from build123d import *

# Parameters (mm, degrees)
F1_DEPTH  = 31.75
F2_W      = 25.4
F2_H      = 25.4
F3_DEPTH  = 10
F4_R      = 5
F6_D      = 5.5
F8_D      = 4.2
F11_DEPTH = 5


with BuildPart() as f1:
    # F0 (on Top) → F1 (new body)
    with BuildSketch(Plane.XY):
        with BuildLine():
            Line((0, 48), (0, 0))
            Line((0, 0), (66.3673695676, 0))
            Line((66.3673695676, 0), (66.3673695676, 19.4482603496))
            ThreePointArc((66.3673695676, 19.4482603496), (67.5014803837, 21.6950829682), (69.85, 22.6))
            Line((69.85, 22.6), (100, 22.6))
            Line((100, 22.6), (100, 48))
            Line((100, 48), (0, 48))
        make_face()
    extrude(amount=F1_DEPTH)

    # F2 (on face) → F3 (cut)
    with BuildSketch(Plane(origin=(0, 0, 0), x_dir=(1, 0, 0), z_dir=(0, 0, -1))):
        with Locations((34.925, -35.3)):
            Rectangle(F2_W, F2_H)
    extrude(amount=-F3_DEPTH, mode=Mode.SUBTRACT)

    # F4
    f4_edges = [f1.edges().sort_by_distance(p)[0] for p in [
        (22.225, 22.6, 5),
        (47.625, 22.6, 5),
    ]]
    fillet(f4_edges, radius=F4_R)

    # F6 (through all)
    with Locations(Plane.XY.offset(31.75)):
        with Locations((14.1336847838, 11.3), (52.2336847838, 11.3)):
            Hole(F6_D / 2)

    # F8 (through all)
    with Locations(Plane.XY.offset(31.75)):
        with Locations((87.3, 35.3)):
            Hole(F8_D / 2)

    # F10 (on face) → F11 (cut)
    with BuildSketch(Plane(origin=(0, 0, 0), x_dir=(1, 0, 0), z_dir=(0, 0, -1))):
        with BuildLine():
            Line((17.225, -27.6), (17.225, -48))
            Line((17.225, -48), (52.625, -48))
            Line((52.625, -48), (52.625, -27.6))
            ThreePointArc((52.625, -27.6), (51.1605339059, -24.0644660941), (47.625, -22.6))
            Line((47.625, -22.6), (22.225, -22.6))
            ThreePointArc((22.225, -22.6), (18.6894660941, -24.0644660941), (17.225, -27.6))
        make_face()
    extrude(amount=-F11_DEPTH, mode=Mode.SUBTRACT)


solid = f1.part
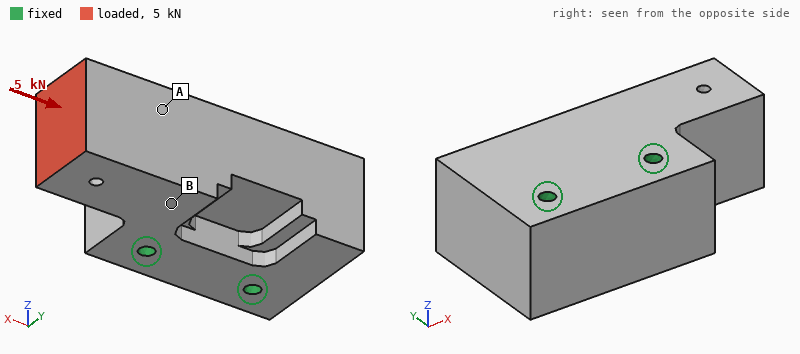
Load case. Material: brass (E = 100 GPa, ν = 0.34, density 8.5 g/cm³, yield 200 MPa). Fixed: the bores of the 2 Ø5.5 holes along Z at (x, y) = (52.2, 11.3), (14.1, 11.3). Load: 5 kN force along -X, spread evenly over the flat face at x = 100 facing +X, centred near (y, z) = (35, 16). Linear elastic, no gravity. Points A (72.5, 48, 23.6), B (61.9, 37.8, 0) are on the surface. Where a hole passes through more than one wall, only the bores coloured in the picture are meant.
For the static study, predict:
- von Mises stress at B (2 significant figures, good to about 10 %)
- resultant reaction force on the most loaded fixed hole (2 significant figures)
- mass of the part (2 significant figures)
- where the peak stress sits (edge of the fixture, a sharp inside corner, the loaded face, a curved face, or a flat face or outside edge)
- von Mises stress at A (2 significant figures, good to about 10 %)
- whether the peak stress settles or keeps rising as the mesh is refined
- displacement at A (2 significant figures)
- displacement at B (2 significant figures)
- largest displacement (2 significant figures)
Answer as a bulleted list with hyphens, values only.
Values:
- 2.9 MPa
- 3.9 kN
- 1.0 kg
- edge of the fixture
- 7.7 MPa
- keeps rising
- 8.0 µm
- 6.4 µm
- 14 µm
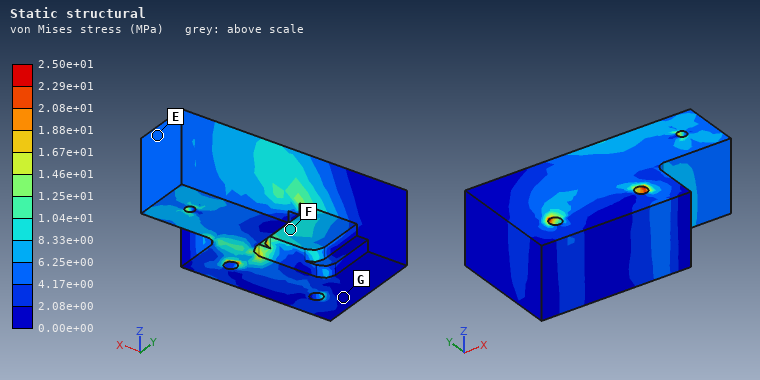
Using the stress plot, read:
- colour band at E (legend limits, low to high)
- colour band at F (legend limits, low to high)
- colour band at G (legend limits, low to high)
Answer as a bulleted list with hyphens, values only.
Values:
- 4.17e+00 to 6.25e+00 MPa
- 8.33e+00 to 1.04e+01 MPa
- 0.00e+00 to 2.08e+00 MPa
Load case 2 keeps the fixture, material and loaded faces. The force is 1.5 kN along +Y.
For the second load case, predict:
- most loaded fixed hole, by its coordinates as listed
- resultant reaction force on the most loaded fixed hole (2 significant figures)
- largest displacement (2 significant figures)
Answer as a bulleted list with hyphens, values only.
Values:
- (52.2, 11.3)
- 3.3 kN
- 19 µm
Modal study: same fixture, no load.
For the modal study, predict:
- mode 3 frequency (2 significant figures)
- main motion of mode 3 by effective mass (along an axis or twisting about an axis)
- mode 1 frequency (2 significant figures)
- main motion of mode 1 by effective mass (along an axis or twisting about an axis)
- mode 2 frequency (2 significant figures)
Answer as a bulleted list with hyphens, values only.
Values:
- 7200 Hz
- along Z
- 3900 Hz
- along Z
- 4600 Hz
